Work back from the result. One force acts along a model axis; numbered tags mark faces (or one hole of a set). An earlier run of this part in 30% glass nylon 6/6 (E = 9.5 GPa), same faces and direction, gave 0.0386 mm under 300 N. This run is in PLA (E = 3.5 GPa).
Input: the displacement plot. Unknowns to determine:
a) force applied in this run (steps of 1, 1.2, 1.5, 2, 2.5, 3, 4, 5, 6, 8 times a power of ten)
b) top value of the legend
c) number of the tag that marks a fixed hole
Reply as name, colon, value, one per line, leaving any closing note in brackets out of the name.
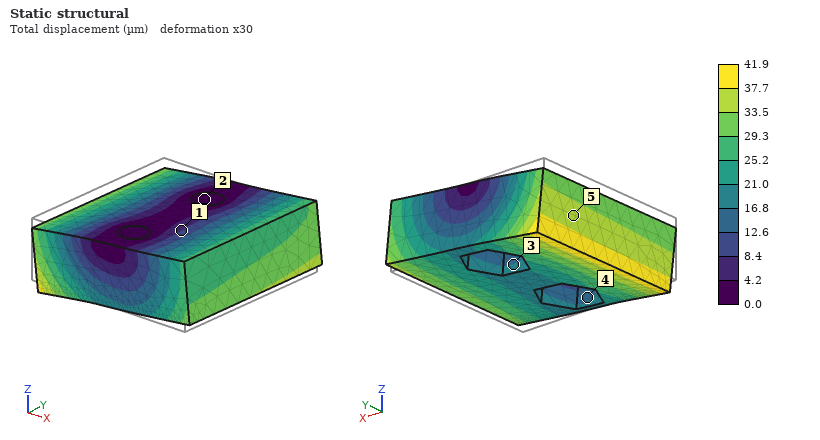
force applied in this run: 120 N
top value of the legend: 41.9 µm
number of the tag that marks a fixed hole: 2
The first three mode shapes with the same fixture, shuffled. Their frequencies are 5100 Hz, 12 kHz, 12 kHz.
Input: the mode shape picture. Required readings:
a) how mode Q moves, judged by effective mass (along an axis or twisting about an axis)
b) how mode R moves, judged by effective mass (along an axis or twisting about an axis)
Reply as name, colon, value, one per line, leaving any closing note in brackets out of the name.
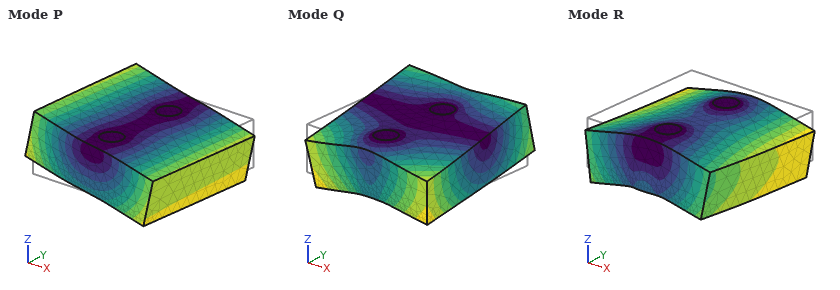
how mode Q moves, judged by effective mass: along Y
how mode R moves, judged by effective mass: along Z
